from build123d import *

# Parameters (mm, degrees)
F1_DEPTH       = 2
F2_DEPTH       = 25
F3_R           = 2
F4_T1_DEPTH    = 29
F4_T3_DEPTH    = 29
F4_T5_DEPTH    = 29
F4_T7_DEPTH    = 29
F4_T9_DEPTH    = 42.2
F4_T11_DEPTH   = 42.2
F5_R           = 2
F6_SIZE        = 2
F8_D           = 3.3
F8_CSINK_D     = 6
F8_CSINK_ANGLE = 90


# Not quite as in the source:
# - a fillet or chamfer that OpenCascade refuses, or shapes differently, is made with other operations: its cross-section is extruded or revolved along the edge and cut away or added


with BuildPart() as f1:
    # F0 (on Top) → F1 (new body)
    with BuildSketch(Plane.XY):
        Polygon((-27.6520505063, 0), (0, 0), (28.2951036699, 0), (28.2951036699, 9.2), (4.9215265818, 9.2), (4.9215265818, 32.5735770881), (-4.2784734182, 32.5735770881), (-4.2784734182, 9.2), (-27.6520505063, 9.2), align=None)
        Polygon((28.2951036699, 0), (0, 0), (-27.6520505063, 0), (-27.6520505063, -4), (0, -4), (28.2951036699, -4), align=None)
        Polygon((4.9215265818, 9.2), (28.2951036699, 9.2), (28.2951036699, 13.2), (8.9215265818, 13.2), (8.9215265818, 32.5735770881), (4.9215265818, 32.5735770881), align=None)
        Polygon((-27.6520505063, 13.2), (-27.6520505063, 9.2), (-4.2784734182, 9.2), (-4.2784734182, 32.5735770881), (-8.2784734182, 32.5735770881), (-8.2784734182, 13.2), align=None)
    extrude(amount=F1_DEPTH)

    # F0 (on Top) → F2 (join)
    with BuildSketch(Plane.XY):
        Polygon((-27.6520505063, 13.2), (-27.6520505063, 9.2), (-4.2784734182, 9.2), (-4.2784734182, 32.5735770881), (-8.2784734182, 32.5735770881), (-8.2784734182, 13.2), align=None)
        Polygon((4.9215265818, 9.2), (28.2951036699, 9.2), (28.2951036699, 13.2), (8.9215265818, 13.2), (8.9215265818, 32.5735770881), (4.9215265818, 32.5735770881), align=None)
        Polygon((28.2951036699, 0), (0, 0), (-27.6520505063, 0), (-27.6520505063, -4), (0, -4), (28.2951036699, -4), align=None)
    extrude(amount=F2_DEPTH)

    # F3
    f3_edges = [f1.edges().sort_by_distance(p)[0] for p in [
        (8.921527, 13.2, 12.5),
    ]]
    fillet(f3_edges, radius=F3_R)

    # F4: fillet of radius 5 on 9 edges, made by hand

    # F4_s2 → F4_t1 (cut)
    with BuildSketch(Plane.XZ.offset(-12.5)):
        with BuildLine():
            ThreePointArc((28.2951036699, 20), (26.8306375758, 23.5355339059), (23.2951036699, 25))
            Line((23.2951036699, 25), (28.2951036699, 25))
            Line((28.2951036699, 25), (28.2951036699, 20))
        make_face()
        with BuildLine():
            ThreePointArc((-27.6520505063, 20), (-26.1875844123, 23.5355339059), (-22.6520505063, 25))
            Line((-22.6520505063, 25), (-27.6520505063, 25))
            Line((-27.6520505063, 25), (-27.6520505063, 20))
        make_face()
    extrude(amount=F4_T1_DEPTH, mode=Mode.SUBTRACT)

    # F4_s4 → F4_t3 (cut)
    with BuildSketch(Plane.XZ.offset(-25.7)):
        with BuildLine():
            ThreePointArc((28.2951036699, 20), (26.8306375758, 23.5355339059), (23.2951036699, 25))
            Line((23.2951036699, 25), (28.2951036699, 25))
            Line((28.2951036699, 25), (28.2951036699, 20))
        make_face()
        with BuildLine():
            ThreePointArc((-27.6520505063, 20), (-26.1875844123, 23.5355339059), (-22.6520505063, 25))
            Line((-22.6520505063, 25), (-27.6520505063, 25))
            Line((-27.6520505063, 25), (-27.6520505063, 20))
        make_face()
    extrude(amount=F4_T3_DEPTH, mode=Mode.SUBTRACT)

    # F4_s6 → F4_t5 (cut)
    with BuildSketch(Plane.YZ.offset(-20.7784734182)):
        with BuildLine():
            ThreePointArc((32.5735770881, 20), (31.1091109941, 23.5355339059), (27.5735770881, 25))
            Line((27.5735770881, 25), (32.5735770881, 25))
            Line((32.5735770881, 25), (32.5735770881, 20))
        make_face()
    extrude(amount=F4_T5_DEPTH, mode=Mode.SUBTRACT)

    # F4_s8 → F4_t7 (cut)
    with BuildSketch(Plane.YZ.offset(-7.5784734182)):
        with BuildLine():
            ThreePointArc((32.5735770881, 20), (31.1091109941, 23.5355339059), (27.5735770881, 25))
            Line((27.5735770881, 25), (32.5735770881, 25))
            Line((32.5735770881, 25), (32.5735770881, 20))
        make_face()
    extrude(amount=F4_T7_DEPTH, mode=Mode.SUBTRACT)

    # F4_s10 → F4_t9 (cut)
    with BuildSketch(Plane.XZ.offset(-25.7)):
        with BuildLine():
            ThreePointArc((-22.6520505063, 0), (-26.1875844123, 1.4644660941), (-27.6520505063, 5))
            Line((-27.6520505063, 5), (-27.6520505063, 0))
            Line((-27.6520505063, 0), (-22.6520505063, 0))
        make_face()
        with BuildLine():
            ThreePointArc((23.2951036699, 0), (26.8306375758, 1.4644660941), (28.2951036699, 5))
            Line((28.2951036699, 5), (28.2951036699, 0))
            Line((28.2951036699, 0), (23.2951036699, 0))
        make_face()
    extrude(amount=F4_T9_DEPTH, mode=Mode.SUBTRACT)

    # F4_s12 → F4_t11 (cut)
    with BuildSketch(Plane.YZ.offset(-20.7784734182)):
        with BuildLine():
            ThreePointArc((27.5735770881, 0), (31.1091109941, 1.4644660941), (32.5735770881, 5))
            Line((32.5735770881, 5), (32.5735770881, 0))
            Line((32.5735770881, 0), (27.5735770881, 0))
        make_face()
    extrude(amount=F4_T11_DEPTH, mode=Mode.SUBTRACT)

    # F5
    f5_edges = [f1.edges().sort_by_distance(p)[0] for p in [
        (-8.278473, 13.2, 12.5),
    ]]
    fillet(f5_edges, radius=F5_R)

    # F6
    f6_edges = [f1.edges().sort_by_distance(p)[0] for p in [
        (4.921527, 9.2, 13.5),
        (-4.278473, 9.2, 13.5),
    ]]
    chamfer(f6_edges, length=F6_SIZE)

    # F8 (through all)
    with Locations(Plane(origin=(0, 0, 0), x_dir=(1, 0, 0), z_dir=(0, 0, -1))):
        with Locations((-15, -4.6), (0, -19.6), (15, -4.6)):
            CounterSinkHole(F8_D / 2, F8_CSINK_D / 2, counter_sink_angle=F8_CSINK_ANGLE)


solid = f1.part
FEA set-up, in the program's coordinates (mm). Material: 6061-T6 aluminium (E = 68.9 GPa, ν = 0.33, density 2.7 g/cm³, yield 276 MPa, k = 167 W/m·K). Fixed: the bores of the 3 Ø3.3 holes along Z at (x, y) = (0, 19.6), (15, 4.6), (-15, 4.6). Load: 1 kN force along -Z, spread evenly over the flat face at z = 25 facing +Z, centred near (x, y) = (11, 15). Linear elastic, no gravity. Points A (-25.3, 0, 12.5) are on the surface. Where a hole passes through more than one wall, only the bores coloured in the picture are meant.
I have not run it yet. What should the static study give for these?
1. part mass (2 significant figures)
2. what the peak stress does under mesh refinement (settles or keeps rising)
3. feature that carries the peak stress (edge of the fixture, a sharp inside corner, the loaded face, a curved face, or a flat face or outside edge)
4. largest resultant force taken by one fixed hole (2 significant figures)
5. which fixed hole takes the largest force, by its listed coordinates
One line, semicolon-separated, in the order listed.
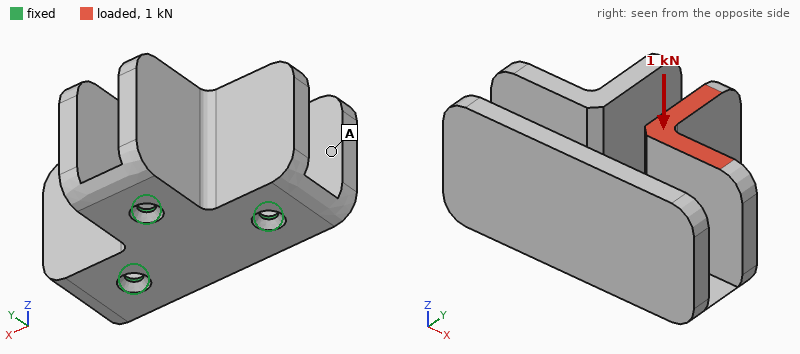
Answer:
41 g; keeps rising; edge of the fixture; 600 N; (0, 19.6)
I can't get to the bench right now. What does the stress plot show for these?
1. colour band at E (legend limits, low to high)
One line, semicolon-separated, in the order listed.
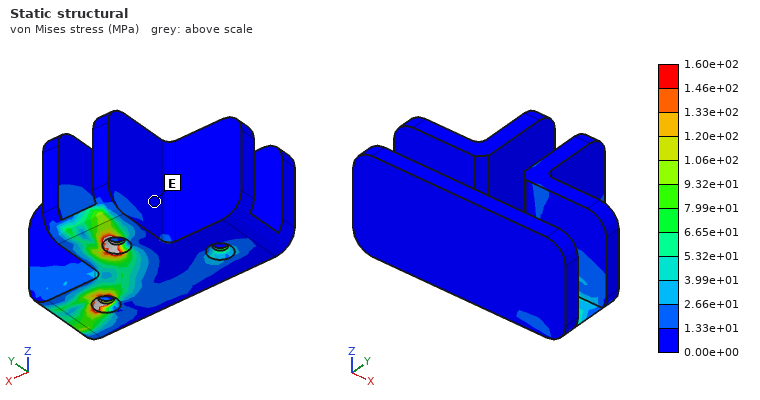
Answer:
0.00e+00 to 1.33e+01 MPa
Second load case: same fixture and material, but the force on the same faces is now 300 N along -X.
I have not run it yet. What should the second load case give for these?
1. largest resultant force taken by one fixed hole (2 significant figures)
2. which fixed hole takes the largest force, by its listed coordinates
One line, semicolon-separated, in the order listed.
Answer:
390 N; (15, 4.6)
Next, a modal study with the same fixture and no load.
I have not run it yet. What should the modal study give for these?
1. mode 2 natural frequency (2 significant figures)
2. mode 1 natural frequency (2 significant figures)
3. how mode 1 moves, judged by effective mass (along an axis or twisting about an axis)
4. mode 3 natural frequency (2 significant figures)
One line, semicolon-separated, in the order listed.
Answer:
2200 Hz; 1500 Hz; along Y; 2600 Hz
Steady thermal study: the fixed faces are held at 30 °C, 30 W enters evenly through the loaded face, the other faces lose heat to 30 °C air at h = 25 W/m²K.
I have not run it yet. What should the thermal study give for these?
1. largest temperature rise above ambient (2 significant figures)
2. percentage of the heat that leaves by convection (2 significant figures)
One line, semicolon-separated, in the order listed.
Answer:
46 K; 9.1 %
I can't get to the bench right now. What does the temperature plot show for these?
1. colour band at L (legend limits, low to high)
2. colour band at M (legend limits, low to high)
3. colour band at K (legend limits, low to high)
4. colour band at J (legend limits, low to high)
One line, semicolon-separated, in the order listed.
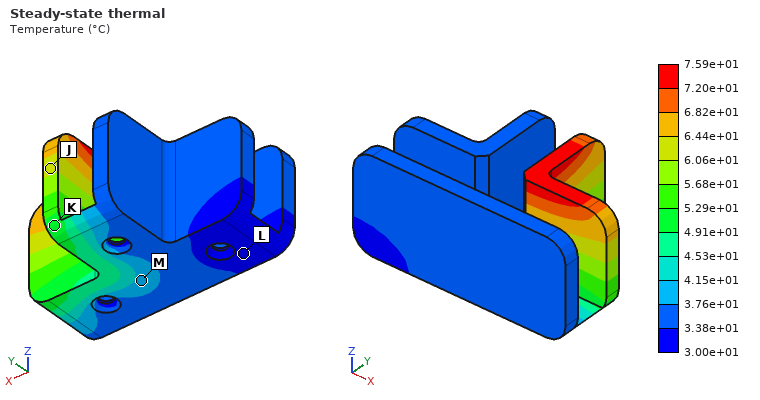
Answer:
3.00e+01 to 3.38e+01 °C; 3.76e+01 to 4.15e+01 °C; 4.91e+01 to 5.29e+01 °C; 6.06e+01 to 6.44e+01 °C
